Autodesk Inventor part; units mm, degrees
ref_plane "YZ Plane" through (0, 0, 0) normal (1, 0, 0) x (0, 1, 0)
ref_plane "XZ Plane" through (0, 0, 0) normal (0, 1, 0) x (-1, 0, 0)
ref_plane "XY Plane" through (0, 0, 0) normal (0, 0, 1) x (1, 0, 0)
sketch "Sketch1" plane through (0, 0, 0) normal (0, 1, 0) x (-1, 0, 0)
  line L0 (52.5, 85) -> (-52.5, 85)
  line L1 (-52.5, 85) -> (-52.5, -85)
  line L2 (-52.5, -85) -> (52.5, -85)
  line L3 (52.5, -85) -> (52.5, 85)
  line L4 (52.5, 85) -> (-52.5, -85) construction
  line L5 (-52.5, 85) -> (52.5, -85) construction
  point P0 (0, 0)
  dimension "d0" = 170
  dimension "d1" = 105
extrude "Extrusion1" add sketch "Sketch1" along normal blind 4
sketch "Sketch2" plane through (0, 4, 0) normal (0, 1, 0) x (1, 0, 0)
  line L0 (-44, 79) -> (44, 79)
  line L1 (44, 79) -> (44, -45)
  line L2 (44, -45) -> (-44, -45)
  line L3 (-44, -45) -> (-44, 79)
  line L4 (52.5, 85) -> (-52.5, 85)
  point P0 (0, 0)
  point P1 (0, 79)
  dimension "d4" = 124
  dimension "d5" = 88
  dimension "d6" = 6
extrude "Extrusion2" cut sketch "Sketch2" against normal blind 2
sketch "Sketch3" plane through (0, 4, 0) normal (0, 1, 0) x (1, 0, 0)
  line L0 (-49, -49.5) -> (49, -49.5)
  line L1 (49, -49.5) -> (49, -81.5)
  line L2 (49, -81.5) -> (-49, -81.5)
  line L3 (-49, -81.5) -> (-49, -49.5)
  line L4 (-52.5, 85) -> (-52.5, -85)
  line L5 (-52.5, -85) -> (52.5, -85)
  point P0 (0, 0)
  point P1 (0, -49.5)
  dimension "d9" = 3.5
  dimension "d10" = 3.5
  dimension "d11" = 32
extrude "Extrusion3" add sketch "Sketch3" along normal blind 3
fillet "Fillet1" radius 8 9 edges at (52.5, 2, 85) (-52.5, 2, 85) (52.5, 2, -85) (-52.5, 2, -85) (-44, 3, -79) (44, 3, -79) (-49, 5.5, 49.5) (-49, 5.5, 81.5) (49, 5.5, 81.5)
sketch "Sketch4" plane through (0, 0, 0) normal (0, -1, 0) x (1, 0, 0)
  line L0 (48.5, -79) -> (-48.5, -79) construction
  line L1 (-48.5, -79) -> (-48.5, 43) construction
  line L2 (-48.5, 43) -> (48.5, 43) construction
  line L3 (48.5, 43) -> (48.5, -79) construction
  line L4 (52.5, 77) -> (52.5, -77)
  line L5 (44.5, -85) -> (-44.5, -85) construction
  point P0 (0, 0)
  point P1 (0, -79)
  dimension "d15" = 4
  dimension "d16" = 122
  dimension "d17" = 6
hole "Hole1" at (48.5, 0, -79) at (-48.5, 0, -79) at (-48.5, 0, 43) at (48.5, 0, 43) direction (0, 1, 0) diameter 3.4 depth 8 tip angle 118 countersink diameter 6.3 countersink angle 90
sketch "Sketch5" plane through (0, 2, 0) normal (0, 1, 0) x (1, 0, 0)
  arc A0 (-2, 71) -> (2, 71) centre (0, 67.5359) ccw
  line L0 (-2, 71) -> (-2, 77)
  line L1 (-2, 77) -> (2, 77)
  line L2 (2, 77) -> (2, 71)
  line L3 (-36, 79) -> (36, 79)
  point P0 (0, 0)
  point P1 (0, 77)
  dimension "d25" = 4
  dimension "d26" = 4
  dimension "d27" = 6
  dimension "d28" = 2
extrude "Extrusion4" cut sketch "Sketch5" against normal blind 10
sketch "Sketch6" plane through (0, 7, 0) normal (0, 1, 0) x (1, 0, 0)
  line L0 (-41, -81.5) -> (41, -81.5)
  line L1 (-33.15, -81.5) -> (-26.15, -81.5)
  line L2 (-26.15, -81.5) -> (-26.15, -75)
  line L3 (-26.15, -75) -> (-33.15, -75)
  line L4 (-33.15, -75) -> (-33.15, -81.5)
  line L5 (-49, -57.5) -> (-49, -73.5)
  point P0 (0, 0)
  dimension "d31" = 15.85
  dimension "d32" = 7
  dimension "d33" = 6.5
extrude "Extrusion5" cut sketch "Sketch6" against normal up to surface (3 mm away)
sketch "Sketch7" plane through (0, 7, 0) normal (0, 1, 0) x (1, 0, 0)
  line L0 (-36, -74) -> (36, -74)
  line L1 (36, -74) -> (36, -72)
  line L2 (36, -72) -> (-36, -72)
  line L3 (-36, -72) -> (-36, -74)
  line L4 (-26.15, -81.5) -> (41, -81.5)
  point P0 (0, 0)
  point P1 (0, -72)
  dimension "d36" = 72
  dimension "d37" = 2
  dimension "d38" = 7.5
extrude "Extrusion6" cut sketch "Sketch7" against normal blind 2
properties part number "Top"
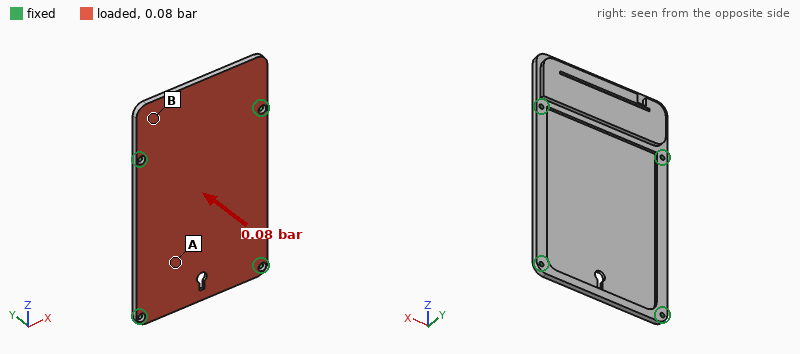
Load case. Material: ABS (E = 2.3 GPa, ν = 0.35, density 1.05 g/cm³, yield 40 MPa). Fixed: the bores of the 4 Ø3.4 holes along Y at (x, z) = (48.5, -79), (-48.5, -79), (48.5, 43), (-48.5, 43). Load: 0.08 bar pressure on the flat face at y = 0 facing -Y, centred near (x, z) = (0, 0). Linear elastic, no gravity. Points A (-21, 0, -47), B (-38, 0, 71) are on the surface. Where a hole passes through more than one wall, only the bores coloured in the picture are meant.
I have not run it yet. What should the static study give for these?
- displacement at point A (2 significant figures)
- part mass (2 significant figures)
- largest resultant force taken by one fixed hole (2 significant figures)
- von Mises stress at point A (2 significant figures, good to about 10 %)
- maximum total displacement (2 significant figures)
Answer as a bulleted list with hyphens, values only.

- 1.5 mm
- 61 g
- 74 N
- 3.3 MPa
- 2.2 mm
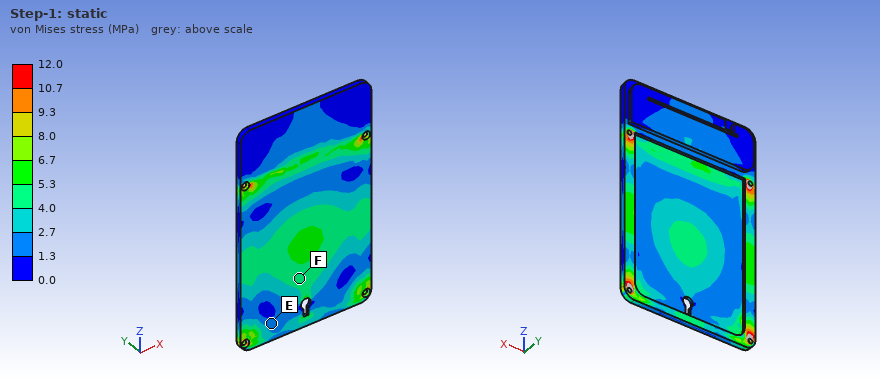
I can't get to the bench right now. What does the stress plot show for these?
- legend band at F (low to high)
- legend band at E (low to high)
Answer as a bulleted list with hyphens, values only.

- 4.0 to 5.3 MPa
- 1.3 to 2.7 MPa
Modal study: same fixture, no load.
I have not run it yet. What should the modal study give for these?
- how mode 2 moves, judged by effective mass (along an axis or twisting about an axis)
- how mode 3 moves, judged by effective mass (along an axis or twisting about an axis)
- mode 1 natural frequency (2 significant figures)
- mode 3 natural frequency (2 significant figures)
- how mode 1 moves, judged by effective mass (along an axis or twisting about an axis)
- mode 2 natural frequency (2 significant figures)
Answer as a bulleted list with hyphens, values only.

- along Y
- twisting about Z
- 230 Hz
- 370 Hz
- twisting about X
- 270 Hz
